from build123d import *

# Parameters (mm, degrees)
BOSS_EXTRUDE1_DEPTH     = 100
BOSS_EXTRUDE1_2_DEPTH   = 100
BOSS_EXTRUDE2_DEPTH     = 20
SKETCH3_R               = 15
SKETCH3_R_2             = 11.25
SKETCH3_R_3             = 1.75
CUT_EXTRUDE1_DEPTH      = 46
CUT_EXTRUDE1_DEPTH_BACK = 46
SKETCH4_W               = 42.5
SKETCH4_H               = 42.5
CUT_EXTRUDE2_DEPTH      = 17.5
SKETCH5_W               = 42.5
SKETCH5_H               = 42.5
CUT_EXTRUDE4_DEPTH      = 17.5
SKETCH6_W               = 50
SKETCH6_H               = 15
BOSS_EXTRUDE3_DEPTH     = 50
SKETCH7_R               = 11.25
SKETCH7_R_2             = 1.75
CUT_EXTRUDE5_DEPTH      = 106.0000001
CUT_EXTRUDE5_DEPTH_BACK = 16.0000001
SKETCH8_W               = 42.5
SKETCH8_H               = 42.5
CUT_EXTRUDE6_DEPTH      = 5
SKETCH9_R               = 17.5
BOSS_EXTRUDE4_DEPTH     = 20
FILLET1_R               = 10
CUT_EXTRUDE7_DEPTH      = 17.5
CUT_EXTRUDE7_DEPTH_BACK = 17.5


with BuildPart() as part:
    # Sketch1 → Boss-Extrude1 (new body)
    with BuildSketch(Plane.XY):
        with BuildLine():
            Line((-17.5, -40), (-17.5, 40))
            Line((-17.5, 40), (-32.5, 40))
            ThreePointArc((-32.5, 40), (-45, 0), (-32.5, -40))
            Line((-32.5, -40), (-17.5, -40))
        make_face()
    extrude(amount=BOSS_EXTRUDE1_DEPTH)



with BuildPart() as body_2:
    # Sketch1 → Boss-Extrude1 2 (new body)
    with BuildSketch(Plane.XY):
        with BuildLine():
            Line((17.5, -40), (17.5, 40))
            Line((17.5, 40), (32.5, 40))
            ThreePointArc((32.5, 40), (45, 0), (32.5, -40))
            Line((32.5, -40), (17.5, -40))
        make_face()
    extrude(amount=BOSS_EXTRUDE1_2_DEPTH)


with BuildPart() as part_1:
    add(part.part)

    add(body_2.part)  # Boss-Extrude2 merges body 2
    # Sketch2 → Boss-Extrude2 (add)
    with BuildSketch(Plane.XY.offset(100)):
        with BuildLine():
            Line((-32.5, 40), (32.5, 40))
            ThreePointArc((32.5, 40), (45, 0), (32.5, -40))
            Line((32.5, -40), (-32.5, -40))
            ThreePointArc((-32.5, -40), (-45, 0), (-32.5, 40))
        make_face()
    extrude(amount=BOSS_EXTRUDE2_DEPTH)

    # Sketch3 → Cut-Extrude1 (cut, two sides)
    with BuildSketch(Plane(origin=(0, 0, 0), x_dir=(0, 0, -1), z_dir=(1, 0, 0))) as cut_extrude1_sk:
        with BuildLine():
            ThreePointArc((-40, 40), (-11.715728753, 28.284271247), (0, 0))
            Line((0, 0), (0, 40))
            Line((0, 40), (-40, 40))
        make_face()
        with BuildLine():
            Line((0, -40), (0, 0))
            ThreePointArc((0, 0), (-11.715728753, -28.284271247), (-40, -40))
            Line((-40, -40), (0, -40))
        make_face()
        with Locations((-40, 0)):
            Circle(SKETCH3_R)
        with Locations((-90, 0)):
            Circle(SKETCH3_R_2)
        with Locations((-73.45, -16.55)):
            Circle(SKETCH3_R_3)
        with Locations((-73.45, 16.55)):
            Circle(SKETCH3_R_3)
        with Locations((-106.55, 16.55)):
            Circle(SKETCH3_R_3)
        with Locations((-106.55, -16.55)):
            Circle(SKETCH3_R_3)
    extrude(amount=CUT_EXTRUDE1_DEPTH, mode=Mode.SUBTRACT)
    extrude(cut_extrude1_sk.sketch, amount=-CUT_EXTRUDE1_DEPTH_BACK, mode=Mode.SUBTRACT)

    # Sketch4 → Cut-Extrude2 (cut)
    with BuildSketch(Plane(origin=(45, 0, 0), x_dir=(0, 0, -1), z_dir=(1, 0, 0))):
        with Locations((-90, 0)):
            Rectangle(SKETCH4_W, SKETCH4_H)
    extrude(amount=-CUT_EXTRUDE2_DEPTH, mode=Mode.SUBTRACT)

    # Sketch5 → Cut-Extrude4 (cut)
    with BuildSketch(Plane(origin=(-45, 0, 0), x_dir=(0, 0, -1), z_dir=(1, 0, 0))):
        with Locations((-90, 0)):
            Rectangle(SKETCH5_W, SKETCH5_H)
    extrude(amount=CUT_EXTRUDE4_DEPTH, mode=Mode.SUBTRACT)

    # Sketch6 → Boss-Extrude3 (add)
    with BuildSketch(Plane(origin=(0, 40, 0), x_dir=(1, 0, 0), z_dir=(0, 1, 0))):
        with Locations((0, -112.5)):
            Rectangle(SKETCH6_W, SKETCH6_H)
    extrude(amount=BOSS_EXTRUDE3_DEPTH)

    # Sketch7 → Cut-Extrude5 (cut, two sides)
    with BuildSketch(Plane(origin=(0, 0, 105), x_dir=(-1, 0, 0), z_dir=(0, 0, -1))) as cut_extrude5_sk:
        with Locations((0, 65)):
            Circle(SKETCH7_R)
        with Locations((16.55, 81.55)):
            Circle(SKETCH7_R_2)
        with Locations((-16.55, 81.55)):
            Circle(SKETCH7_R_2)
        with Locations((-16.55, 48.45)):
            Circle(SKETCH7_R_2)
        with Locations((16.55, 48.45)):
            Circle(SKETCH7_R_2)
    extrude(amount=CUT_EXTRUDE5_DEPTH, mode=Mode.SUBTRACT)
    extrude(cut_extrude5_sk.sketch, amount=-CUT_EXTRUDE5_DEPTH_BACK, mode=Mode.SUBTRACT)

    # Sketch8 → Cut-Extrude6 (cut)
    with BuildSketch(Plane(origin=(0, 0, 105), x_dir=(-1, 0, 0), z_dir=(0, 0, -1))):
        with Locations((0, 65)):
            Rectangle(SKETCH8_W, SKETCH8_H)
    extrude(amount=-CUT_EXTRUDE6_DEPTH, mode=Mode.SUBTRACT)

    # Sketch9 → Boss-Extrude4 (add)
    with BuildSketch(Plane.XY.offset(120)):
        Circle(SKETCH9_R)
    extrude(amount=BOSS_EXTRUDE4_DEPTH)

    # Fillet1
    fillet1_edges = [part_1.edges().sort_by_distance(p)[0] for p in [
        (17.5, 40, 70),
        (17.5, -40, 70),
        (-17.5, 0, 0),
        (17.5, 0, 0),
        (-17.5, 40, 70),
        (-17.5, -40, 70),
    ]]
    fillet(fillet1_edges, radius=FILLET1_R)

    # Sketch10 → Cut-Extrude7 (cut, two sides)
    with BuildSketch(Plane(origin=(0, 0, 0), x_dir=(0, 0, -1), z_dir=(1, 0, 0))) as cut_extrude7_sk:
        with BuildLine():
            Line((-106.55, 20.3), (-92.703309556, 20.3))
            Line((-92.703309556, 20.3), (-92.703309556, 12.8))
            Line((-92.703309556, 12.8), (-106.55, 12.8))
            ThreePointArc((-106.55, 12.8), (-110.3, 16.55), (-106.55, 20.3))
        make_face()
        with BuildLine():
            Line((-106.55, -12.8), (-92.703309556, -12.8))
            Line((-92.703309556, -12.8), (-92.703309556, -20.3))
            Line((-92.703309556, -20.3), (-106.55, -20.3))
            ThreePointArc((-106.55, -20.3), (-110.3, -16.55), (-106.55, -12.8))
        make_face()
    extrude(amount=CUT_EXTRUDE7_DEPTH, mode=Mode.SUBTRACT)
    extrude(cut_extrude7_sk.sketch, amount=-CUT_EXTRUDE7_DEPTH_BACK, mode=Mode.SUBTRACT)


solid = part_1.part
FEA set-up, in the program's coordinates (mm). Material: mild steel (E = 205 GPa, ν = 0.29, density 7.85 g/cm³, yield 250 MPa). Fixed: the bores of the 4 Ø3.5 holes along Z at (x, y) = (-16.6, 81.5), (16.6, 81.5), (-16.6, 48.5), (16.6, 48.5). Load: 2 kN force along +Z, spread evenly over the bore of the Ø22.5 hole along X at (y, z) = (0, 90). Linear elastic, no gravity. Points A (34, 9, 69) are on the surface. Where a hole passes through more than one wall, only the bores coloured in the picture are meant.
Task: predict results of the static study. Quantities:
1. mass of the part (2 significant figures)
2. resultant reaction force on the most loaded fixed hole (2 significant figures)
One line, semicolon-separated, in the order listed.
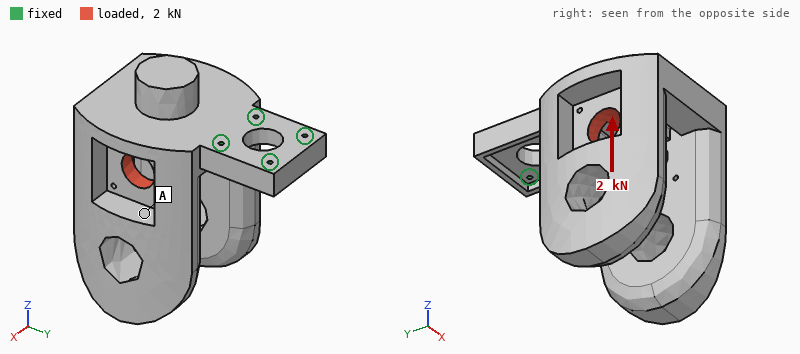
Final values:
3.2 kg; 1.6 kN
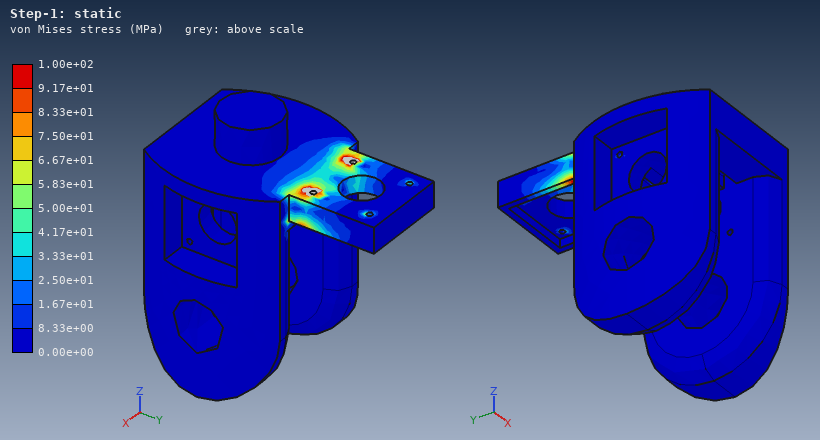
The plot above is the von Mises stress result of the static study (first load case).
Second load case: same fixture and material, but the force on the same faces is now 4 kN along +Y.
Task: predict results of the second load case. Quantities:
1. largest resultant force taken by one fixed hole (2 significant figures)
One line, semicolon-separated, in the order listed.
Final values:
1.6 kN
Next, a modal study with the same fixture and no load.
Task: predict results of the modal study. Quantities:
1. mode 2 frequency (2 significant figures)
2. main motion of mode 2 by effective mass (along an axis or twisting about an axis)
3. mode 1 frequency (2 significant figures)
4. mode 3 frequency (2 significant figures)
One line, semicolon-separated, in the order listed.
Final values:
600 Hz; along X; 330 Hz; 970 Hz
